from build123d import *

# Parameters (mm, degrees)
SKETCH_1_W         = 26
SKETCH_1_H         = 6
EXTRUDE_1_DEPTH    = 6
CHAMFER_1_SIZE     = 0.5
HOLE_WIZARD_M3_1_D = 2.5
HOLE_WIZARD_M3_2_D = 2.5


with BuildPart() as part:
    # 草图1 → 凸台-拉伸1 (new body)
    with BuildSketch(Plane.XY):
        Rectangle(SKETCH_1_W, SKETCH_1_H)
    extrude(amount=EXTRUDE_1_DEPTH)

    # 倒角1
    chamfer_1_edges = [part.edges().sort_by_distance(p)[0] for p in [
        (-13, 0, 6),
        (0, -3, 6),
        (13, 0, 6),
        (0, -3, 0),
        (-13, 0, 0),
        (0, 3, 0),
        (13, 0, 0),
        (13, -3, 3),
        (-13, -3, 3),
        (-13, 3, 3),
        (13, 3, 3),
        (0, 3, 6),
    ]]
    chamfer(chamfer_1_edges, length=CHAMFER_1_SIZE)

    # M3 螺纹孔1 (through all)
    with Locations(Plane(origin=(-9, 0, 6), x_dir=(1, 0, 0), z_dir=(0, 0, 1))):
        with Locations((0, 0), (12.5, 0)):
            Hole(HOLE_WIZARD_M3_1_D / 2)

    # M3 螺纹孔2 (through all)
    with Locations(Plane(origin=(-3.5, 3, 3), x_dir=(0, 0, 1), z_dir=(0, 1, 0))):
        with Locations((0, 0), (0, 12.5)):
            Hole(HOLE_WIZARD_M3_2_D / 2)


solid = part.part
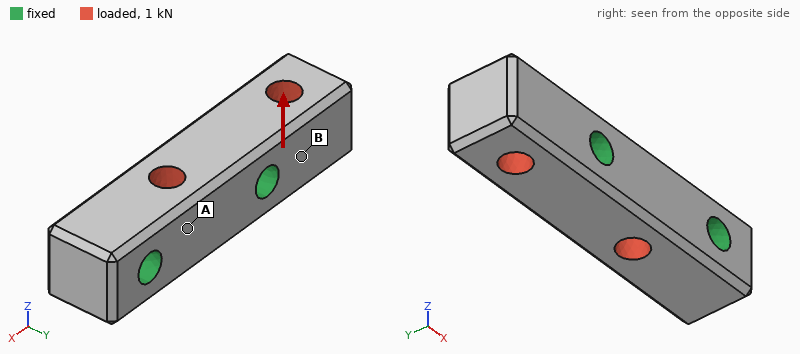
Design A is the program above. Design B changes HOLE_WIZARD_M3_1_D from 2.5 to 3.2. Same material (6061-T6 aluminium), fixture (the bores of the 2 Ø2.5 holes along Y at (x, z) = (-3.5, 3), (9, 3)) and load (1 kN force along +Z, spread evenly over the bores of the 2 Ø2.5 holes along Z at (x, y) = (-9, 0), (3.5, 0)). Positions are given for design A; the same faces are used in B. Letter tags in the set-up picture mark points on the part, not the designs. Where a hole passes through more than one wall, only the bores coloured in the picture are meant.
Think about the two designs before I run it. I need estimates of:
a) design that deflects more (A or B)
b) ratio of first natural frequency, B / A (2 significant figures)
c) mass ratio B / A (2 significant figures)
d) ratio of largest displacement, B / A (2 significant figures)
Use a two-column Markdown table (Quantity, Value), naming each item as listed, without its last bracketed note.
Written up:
| Quantity | Value |
|---|---|
| design that deflects more | B |
| ratio of first natural frequency, B / A | 0.98 |
| mass ratio B / A | 0.95 |
| ratio of largest displacement, B / A | 1.1 |
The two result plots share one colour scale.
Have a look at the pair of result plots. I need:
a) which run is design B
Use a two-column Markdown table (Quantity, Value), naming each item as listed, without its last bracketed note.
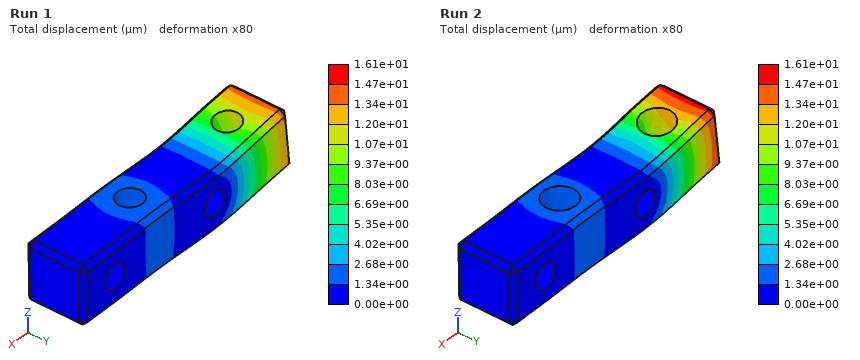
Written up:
| Quantity | Value |
|---|---|
| which run is design B | Run 2 |
